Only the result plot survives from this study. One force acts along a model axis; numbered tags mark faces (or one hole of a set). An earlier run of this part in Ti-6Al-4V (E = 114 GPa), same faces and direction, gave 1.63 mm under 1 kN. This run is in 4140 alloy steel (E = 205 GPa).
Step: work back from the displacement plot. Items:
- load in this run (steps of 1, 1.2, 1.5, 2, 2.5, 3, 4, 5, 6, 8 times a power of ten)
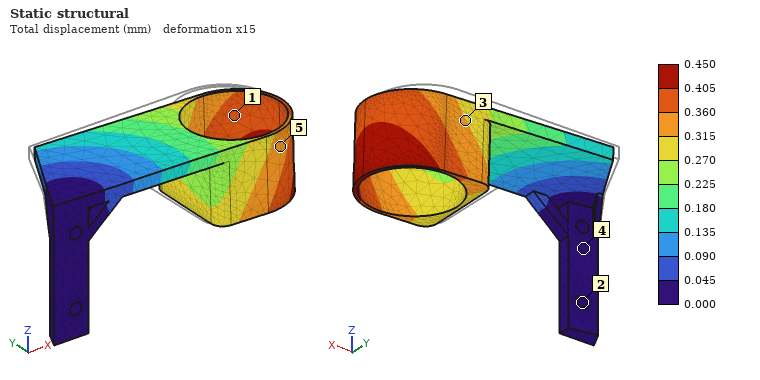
500 N
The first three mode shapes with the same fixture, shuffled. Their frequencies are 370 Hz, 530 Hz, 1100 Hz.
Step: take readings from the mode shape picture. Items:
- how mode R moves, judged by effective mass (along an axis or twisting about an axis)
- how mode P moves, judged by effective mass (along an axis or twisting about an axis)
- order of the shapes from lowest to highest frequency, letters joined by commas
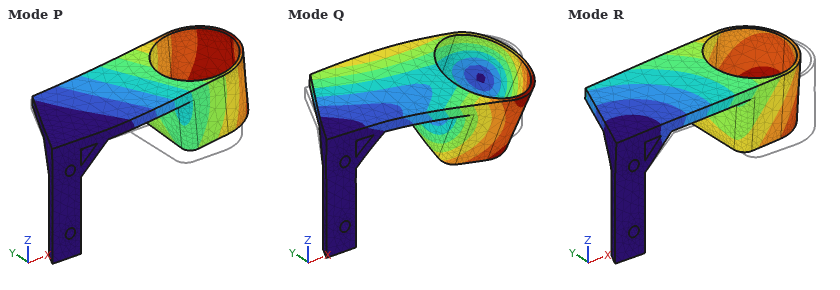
along Y
along Z
P, R, Q
